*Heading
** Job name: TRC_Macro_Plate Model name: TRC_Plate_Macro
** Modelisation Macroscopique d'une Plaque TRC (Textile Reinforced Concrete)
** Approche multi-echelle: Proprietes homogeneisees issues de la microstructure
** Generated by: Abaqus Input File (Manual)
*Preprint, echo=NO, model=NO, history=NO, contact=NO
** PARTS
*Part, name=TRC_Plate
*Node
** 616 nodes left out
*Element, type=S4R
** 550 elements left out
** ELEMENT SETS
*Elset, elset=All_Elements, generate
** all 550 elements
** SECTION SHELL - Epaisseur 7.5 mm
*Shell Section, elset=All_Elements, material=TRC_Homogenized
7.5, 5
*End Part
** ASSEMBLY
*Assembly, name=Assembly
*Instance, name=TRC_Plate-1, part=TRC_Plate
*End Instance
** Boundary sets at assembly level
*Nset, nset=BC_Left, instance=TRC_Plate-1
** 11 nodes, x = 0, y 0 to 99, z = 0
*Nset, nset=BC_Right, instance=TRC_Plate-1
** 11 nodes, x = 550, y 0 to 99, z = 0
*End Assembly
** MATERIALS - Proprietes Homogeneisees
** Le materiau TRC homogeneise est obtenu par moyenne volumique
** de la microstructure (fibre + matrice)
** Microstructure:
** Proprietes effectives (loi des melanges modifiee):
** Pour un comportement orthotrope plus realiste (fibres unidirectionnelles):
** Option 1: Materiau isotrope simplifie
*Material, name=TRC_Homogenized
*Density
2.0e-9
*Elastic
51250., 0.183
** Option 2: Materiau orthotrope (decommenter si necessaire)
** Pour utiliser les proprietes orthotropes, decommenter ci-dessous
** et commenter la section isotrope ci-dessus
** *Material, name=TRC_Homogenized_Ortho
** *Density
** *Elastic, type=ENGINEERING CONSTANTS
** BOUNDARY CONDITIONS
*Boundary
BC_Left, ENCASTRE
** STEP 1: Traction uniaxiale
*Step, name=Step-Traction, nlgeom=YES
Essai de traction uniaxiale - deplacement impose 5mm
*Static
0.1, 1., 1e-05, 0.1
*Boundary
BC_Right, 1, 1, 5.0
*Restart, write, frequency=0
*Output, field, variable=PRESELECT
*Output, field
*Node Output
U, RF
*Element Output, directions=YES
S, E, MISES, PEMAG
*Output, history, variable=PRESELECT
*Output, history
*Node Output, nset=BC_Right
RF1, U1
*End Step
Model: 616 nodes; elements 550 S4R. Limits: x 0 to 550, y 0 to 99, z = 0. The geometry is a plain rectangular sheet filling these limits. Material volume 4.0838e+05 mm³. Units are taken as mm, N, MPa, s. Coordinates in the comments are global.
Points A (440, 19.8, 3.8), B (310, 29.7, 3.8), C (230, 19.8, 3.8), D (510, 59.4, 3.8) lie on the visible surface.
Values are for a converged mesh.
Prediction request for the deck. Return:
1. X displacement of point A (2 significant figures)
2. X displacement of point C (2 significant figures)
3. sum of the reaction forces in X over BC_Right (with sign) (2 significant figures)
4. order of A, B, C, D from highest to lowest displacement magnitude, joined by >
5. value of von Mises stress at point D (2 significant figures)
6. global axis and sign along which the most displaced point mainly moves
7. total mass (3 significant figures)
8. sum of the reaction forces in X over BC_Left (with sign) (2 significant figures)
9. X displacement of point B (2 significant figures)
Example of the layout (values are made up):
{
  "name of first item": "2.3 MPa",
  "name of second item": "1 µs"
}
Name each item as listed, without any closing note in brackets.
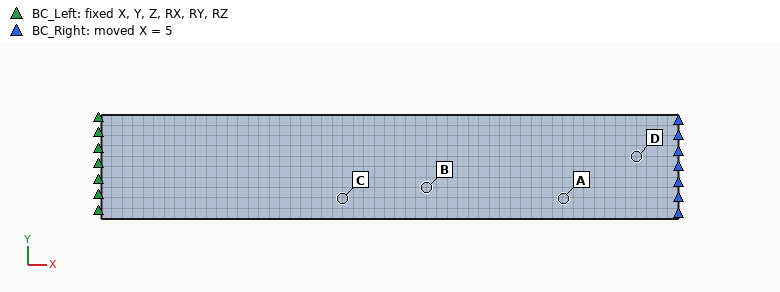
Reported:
{
  "X displacement of point A": "4.0 mm",
  "X displacement of point C": "2.1 mm",
  "sum of the reaction forces in X over BC_Right (with sign)": "3.5e+05 N",
  "order of A, B, C, D from highest to lowest displacement magnitude, joined by >": "D > A > B > C",
  "value of von Mises stress at point D": "470 MPa",
  "global axis and sign along which the most displaced point mainly moves": "+X",
  "total mass": "0.817 kg",
  "sum of the reaction forces in X over BC_Left (with sign)": "-3.5e+05 N",
  "X displacement of point B": "2.8 mm"
}
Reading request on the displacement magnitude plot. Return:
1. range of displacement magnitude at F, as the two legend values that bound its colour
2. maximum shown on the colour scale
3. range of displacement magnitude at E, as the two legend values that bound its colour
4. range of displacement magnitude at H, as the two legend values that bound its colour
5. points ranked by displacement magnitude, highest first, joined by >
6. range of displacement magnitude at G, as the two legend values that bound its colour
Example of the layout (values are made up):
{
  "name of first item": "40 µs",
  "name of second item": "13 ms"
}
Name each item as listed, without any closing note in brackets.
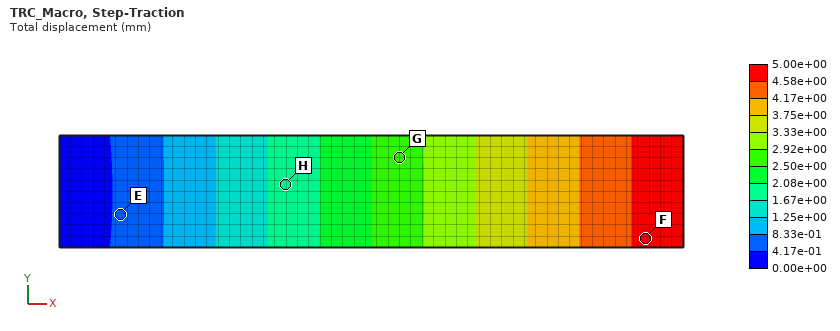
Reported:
{
  "range of displacement magnitude at F, as the two legend values that bound its colour": "4.58e+00 to 5.00e+00 mm",
  "maximum shown on the colour scale": "5.00e+00 mm",
  "range of displacement magnitude at E, as the two legend values that bound its colour": "4.17e-01 to 8.33e-01 mm",
  "range of displacement magnitude at H, as the two legend values that bound its colour": "1.67e+00 to 2.08e+00 mm",
  "points ranked by displacement magnitude, highest first, joined by >": "F > G > H > E",
  "range of displacement magnitude at G, as the two legend values that bound its colour": "2.50e+00 to 2.92e+00 mm"
}
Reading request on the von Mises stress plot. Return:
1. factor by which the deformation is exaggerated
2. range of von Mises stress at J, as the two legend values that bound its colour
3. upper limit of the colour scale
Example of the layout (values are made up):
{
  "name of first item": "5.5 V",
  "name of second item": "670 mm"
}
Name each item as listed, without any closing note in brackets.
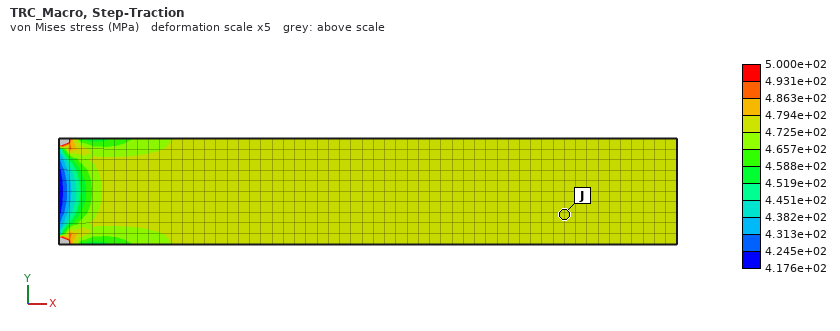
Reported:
{
  "factor by which the deformation is exaggerated": "5",
  "range of von Mises stress at J, as the two legend values that bound its colour": "4.725e+02 to 4.794e+02 MPa",
  "upper limit of the colour scale": "5.000e+02 MPa"
}
